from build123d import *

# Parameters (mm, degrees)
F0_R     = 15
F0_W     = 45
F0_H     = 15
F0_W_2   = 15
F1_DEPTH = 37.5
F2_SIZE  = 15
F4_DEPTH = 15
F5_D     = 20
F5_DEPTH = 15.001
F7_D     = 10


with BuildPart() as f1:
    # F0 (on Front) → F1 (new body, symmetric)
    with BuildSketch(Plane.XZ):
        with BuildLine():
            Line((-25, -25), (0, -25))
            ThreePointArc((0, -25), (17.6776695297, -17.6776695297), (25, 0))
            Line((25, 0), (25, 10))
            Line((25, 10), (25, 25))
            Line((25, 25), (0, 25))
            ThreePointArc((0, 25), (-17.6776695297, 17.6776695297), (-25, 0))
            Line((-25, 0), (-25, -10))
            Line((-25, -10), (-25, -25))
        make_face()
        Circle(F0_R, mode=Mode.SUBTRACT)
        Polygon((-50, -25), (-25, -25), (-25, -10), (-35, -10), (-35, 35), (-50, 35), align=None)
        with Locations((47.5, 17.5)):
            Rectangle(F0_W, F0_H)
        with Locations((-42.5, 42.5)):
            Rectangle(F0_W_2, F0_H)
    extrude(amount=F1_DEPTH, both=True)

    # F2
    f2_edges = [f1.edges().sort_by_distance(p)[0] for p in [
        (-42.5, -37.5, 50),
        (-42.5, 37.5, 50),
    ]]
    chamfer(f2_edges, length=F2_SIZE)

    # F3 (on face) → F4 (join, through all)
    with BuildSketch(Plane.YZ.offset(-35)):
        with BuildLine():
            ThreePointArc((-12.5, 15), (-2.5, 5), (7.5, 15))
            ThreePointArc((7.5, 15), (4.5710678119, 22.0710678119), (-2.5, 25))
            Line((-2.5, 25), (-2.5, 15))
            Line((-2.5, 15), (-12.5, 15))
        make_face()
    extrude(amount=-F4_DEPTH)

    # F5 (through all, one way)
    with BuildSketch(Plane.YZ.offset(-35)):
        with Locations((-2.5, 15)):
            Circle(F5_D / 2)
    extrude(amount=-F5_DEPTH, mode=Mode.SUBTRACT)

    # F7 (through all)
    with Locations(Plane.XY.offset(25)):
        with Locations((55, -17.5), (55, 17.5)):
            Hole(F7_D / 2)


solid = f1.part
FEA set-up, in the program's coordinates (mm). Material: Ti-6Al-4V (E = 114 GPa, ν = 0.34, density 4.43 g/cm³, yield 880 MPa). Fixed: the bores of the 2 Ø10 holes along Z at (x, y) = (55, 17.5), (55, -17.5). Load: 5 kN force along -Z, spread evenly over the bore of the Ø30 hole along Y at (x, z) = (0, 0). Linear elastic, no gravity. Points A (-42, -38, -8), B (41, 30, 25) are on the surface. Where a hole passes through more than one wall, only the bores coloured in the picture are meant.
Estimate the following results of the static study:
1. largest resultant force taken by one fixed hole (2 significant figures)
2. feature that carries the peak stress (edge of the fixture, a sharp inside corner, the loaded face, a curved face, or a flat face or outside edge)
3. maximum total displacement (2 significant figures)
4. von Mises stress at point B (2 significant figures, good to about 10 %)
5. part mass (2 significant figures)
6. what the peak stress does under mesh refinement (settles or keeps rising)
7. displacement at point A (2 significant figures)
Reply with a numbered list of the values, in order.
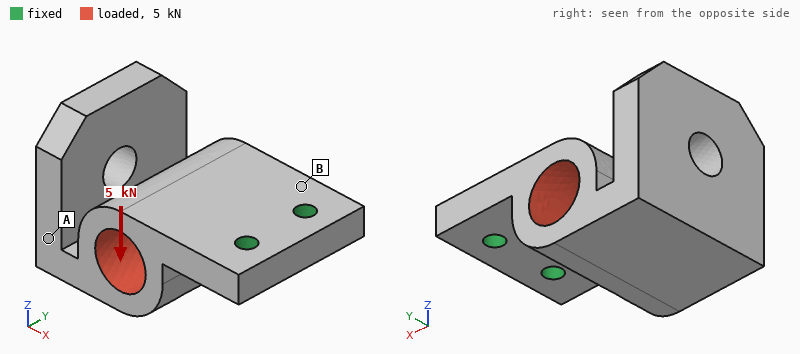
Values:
1. 2.5 kN
2. edge of the fixture
3. 0.29 mm
4. 62 MPa
5. 1.1 kg
6. keeps rising
7. 0.25 mm
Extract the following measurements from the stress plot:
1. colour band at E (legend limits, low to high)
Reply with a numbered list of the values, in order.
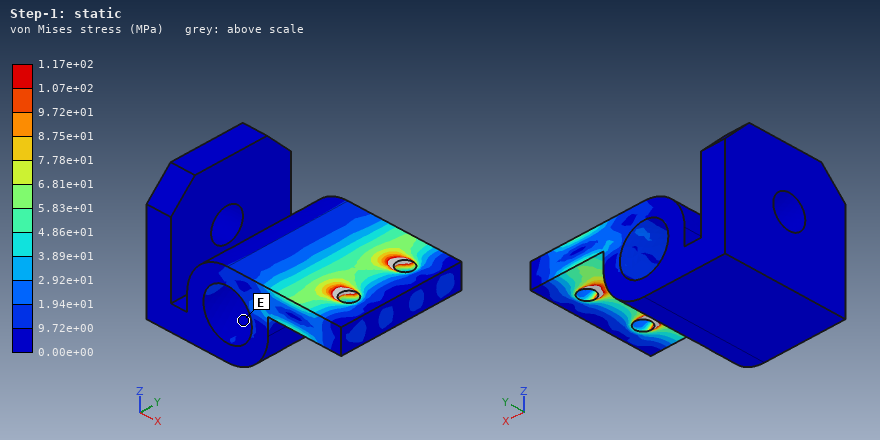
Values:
1. 0.00e+00 to 9.72e+00 MPa
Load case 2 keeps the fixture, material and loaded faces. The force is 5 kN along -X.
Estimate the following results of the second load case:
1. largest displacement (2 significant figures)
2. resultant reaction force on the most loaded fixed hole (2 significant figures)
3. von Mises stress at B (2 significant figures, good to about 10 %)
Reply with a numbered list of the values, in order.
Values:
1. 0.14 mm
2. 2.5 kN
3. 24 MPa
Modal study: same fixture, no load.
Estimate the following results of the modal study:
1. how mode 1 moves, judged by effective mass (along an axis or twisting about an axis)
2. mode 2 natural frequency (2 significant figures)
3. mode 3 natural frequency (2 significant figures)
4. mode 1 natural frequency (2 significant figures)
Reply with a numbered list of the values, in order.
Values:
1. along Z
2. 1800 Hz
3. 1800 Hz
4. 650 Hz
